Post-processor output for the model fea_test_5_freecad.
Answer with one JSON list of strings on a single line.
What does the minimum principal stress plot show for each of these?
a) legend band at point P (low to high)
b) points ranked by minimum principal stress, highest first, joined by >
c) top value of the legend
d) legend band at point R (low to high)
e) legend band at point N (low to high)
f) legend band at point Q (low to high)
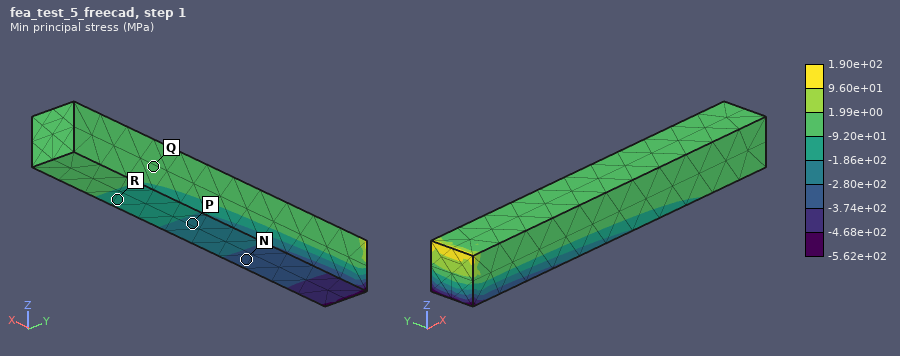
["-2.80e+02 to -1.86e+02 MPa", "Q > R > P > N", "1.90e+02 MPa", "-1.86e+02 to -9.20e+01 MPa", "-3.74e+02 to -2.80e+02 MPa", "-9.20e+01 to 1.99e+00 MPa"]
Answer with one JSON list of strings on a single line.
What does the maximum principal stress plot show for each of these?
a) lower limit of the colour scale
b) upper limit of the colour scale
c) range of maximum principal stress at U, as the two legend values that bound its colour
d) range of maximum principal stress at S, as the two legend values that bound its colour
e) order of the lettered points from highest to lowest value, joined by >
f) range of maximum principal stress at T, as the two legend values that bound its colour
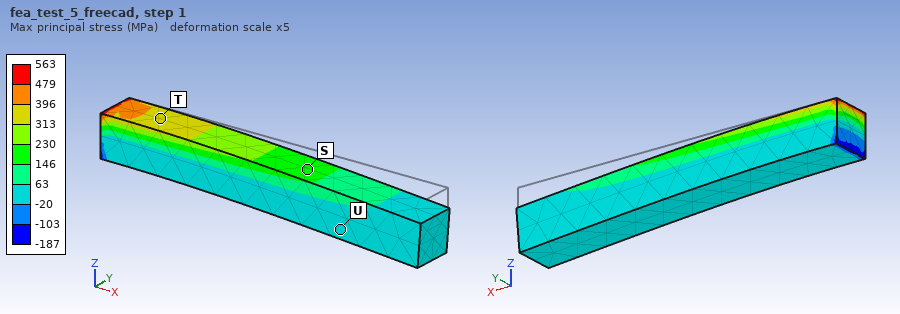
["-187 MPa", "563 MPa", "-20 to 63 MPa", "146 to 230 MPa", "T > S > U", "313 to 396 MPa"]
